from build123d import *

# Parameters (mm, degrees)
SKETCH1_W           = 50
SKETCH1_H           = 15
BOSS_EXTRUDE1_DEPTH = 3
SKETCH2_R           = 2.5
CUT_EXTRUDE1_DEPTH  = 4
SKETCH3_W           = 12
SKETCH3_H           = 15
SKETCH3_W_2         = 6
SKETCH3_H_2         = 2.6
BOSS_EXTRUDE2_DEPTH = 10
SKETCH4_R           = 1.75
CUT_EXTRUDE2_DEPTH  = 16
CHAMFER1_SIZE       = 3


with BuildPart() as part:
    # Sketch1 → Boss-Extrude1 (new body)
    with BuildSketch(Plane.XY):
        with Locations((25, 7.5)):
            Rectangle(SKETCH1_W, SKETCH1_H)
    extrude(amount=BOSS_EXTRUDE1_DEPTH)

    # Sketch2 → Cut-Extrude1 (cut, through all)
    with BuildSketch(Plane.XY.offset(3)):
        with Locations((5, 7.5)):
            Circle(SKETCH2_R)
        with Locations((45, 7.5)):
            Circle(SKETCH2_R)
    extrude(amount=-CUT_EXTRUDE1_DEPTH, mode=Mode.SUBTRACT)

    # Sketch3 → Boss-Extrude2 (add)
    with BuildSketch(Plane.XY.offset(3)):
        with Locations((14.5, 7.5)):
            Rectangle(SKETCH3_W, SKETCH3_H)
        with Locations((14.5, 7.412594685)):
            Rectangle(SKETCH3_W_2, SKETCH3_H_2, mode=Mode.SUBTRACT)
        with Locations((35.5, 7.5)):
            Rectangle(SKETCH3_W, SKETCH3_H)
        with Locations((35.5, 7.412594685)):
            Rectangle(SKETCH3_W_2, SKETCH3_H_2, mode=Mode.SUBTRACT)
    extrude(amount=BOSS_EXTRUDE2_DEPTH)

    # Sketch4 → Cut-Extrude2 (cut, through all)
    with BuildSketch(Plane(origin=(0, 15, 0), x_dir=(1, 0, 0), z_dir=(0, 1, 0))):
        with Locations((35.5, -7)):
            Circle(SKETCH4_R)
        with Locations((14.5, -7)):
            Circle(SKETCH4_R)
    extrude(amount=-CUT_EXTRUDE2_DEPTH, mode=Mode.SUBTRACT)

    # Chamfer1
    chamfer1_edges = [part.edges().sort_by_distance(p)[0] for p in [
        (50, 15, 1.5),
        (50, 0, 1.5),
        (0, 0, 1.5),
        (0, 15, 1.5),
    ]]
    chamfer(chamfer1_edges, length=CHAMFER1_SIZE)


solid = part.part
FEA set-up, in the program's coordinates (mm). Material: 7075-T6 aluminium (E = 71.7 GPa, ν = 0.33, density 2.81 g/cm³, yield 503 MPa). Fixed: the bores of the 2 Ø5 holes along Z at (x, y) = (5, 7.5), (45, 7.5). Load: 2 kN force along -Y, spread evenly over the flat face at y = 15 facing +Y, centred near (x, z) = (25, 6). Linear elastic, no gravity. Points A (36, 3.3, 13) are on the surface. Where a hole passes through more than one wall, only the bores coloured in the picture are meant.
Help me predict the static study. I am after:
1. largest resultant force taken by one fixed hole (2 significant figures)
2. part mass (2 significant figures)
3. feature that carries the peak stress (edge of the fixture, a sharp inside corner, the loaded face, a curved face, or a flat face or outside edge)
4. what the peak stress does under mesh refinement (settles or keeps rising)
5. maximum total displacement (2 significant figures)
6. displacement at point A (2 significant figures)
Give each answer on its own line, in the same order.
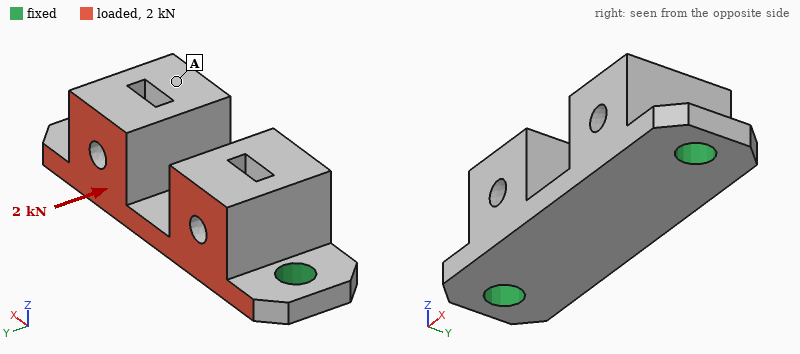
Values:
1.0 kN
14 g
edge of the fixture
keeps rising
47 µm
39 µm
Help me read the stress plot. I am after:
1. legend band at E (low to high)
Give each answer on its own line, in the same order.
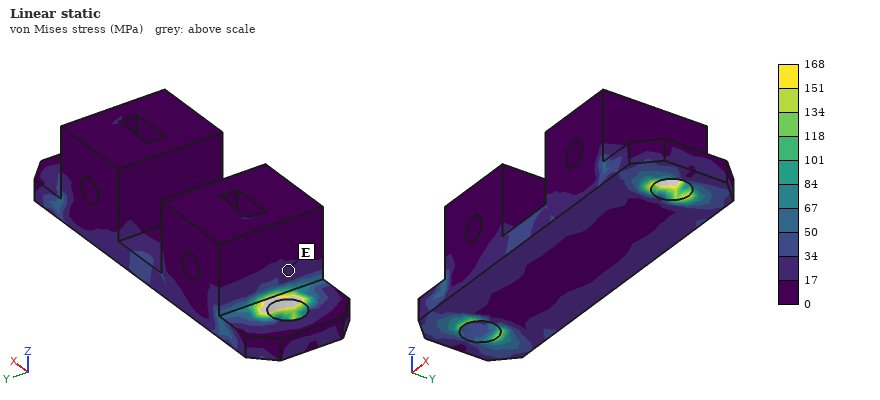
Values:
17 to 34 MPa
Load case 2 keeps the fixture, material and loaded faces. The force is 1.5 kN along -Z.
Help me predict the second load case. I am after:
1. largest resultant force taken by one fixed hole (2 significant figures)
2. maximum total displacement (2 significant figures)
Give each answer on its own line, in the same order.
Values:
750 N
0.11 mm
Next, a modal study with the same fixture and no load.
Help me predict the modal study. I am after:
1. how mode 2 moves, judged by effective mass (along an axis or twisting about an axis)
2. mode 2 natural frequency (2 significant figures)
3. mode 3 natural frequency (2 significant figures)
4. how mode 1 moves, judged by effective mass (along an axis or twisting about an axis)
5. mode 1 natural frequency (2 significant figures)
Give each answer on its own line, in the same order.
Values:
along Y
10 kHz
13 kHz
along Z
6400 Hz
